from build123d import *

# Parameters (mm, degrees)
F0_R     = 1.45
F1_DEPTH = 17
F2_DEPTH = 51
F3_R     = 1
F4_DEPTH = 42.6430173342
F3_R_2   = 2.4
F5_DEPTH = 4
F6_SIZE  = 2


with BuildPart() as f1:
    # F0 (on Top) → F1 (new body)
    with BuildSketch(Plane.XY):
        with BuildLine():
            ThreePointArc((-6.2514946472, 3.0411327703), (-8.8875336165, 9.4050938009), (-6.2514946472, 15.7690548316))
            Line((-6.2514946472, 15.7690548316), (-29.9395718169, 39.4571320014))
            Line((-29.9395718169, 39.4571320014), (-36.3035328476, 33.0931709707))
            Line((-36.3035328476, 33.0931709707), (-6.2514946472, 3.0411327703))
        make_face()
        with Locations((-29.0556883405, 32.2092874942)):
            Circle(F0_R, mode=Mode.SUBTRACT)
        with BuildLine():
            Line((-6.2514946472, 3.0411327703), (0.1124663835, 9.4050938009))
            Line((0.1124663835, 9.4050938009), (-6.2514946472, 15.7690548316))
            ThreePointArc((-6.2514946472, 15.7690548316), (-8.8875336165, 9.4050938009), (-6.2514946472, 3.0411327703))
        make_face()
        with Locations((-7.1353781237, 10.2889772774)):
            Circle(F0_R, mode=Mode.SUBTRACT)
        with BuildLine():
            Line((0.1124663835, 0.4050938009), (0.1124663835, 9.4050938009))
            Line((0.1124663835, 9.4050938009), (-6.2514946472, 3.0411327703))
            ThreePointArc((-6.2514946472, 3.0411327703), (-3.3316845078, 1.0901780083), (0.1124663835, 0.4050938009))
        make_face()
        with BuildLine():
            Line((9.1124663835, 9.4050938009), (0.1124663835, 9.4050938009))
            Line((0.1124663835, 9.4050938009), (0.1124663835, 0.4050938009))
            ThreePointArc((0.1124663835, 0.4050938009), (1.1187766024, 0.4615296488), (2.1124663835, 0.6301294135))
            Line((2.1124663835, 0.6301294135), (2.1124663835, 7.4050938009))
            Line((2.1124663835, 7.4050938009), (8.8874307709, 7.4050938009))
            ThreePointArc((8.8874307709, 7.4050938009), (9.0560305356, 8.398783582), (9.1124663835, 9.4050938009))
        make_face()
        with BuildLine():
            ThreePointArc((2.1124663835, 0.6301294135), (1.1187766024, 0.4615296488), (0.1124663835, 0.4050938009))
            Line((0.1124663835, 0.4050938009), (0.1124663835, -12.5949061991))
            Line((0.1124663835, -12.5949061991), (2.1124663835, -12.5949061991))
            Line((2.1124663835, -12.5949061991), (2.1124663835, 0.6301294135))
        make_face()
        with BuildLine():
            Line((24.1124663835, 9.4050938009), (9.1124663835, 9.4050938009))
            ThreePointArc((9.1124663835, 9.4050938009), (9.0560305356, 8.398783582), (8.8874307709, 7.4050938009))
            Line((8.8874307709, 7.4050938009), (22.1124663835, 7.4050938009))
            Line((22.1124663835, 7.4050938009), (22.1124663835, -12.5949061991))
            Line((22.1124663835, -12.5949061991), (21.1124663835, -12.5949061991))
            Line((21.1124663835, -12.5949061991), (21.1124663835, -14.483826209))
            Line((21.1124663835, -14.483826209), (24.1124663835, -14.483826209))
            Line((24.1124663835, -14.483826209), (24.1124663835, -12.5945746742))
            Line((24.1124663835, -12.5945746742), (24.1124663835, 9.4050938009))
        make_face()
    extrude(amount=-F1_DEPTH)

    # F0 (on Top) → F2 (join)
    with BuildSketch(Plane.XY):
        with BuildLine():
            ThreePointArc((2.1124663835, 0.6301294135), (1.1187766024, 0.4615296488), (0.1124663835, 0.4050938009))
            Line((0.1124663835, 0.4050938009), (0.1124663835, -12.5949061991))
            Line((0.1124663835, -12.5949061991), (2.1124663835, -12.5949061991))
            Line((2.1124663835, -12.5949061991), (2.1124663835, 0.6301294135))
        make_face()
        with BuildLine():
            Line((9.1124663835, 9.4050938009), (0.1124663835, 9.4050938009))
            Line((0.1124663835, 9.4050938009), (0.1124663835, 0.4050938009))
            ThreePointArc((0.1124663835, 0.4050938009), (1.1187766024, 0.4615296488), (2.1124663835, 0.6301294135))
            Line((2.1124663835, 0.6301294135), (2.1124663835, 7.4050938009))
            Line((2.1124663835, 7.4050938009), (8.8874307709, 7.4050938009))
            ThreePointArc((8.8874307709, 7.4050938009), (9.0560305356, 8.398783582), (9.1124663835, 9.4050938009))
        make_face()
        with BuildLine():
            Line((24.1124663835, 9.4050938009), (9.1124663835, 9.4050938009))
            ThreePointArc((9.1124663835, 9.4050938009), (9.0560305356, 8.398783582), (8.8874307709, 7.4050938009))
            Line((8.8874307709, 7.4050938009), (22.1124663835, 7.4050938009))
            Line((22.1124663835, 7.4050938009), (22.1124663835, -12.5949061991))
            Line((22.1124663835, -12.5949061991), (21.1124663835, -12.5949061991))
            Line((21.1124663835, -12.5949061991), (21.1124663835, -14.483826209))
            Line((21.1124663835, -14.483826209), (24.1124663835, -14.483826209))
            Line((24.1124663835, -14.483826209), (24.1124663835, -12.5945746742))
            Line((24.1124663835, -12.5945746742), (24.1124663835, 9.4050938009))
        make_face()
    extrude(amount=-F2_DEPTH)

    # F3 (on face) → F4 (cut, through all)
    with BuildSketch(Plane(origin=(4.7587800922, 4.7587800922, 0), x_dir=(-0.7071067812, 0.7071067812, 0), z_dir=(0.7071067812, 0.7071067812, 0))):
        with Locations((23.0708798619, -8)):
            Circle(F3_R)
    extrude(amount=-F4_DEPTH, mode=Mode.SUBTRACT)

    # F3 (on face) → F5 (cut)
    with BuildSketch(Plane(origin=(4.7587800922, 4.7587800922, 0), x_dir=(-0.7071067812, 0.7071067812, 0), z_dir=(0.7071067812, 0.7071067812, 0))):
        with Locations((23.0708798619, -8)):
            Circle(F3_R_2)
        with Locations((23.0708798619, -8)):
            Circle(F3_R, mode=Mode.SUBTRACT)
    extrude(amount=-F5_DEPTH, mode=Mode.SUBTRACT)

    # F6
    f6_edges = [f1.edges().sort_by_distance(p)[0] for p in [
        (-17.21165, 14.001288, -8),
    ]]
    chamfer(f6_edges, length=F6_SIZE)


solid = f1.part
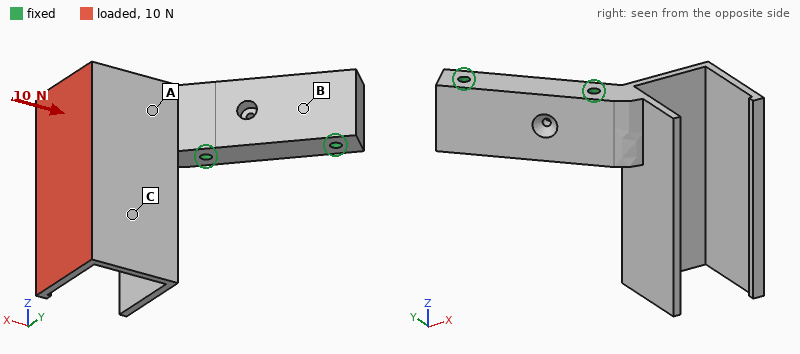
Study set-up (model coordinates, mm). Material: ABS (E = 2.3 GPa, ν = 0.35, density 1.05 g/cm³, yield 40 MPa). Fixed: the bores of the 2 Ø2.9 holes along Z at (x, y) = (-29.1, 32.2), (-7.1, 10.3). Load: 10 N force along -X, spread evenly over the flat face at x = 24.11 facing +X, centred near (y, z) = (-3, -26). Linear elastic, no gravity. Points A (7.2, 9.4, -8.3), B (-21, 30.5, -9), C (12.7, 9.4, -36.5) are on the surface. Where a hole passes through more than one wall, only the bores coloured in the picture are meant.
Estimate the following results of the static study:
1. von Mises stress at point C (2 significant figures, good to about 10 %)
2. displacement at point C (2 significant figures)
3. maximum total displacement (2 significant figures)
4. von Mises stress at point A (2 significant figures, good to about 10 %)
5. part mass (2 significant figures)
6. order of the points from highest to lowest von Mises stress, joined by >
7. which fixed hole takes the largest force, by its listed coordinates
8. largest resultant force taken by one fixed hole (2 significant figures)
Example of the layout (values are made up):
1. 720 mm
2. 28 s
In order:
1. 2.3 MPa
2. 0.20 mm
3. 1.1 mm
4. 3.6 MPa
5. 14 g
6. A > C > B
7. (-7.1, 10.3)
8. 11 N
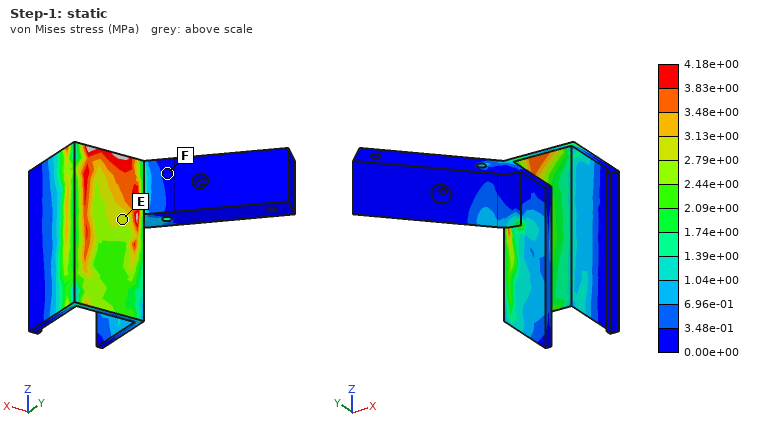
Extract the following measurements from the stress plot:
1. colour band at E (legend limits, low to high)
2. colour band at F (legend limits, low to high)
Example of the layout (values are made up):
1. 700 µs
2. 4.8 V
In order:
1. 2.79e+00 to 3.13e+00 MPa
2. 0.00e+00 to 3.48e-01 MPa
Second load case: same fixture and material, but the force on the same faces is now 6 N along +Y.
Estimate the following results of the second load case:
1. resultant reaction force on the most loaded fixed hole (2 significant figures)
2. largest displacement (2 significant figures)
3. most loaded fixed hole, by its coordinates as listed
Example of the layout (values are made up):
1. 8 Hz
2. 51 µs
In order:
1. 8.1 N
2. 0.94 mm
3. (-7.1, 10.3)
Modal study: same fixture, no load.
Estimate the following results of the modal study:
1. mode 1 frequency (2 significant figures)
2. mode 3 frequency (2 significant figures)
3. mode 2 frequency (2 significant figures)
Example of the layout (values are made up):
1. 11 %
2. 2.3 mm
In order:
1. 250 Hz
2. 750 Hz
3. 480 Hz
